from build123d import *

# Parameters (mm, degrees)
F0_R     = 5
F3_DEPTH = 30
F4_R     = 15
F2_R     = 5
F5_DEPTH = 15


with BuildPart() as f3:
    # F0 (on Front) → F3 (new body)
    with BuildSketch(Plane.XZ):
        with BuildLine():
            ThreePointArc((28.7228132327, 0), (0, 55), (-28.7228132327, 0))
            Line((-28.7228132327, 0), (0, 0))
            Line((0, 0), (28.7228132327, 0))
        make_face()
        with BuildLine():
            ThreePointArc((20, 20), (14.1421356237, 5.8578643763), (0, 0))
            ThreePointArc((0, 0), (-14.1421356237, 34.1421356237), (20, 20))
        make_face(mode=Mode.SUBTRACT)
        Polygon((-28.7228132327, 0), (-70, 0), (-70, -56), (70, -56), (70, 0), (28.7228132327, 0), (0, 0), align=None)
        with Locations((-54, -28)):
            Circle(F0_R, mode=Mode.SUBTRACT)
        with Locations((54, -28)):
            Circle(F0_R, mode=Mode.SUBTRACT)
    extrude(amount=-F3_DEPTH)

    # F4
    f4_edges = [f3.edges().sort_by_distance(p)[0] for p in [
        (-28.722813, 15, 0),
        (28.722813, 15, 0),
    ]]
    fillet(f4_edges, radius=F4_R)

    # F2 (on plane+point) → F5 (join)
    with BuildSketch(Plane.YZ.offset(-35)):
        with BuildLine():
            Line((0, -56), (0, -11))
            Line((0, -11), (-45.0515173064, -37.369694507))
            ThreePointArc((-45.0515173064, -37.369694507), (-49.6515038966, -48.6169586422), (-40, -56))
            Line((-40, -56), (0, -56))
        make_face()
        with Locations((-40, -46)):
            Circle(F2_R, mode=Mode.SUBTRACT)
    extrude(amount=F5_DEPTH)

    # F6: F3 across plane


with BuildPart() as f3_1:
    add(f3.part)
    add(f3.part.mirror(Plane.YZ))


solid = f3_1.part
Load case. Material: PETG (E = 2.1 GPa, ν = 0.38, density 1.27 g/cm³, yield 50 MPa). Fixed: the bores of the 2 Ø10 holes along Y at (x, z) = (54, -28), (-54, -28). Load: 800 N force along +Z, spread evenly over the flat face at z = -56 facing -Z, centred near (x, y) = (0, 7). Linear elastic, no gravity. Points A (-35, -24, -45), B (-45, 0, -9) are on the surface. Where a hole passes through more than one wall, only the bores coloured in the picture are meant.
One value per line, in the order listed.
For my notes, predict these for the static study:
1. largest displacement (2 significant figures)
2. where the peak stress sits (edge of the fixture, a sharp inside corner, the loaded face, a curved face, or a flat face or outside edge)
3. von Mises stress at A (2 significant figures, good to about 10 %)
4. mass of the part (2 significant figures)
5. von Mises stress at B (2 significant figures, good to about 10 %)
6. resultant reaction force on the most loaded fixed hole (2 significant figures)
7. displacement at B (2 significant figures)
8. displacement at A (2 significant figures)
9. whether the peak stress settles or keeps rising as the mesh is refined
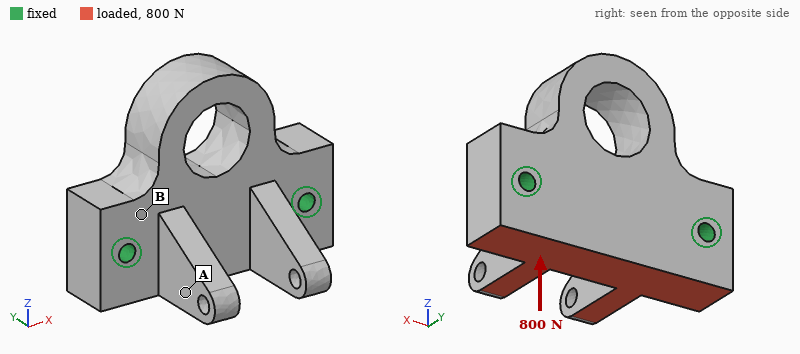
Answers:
51 µm
edge of the fixture
0.21 MPa
430 g
0.54 MPa
400 N
8.4 µm
32 µm
keeps rising
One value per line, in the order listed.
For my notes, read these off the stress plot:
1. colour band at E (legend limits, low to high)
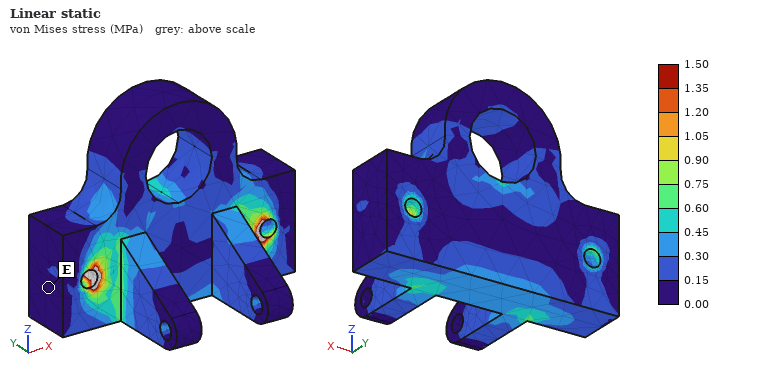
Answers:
0.00 to 0.15 MPa
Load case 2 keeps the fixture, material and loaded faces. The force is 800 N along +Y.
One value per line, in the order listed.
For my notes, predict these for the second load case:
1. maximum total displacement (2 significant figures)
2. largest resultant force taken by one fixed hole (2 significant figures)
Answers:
0.10 mm
400 N
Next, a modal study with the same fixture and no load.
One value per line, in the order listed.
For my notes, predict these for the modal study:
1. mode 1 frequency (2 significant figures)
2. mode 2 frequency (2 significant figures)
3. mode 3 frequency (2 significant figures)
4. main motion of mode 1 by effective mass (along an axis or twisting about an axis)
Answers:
840 Hz
1300 Hz
1400 Hz
along Y
